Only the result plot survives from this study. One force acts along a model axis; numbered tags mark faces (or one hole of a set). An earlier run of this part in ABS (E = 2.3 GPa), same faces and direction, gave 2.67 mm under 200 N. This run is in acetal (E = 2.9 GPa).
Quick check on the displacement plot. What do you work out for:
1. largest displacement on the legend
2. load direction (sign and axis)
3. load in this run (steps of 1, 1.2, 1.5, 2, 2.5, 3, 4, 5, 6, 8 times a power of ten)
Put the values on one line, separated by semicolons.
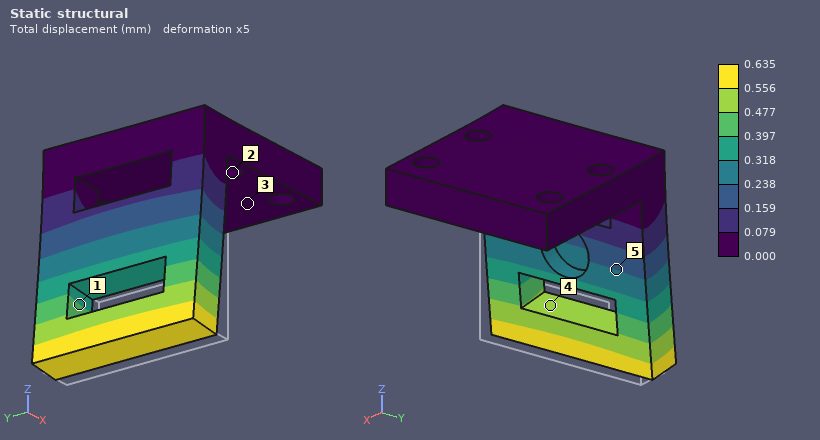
0.635 mm; -X; 60 N
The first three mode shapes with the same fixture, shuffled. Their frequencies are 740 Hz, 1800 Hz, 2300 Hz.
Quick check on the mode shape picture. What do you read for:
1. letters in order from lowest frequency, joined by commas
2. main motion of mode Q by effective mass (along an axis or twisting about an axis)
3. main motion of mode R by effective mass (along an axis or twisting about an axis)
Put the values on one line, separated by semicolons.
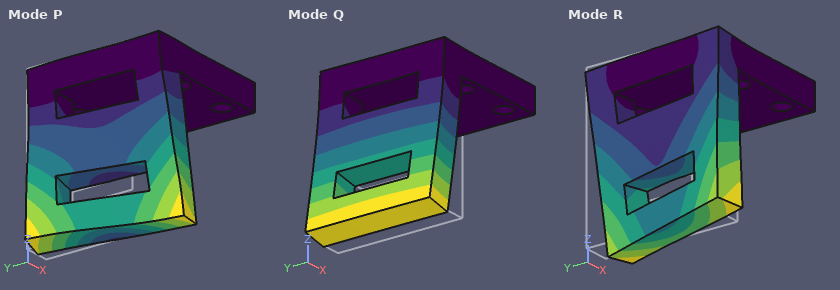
Q, R, P; along X; along Y
